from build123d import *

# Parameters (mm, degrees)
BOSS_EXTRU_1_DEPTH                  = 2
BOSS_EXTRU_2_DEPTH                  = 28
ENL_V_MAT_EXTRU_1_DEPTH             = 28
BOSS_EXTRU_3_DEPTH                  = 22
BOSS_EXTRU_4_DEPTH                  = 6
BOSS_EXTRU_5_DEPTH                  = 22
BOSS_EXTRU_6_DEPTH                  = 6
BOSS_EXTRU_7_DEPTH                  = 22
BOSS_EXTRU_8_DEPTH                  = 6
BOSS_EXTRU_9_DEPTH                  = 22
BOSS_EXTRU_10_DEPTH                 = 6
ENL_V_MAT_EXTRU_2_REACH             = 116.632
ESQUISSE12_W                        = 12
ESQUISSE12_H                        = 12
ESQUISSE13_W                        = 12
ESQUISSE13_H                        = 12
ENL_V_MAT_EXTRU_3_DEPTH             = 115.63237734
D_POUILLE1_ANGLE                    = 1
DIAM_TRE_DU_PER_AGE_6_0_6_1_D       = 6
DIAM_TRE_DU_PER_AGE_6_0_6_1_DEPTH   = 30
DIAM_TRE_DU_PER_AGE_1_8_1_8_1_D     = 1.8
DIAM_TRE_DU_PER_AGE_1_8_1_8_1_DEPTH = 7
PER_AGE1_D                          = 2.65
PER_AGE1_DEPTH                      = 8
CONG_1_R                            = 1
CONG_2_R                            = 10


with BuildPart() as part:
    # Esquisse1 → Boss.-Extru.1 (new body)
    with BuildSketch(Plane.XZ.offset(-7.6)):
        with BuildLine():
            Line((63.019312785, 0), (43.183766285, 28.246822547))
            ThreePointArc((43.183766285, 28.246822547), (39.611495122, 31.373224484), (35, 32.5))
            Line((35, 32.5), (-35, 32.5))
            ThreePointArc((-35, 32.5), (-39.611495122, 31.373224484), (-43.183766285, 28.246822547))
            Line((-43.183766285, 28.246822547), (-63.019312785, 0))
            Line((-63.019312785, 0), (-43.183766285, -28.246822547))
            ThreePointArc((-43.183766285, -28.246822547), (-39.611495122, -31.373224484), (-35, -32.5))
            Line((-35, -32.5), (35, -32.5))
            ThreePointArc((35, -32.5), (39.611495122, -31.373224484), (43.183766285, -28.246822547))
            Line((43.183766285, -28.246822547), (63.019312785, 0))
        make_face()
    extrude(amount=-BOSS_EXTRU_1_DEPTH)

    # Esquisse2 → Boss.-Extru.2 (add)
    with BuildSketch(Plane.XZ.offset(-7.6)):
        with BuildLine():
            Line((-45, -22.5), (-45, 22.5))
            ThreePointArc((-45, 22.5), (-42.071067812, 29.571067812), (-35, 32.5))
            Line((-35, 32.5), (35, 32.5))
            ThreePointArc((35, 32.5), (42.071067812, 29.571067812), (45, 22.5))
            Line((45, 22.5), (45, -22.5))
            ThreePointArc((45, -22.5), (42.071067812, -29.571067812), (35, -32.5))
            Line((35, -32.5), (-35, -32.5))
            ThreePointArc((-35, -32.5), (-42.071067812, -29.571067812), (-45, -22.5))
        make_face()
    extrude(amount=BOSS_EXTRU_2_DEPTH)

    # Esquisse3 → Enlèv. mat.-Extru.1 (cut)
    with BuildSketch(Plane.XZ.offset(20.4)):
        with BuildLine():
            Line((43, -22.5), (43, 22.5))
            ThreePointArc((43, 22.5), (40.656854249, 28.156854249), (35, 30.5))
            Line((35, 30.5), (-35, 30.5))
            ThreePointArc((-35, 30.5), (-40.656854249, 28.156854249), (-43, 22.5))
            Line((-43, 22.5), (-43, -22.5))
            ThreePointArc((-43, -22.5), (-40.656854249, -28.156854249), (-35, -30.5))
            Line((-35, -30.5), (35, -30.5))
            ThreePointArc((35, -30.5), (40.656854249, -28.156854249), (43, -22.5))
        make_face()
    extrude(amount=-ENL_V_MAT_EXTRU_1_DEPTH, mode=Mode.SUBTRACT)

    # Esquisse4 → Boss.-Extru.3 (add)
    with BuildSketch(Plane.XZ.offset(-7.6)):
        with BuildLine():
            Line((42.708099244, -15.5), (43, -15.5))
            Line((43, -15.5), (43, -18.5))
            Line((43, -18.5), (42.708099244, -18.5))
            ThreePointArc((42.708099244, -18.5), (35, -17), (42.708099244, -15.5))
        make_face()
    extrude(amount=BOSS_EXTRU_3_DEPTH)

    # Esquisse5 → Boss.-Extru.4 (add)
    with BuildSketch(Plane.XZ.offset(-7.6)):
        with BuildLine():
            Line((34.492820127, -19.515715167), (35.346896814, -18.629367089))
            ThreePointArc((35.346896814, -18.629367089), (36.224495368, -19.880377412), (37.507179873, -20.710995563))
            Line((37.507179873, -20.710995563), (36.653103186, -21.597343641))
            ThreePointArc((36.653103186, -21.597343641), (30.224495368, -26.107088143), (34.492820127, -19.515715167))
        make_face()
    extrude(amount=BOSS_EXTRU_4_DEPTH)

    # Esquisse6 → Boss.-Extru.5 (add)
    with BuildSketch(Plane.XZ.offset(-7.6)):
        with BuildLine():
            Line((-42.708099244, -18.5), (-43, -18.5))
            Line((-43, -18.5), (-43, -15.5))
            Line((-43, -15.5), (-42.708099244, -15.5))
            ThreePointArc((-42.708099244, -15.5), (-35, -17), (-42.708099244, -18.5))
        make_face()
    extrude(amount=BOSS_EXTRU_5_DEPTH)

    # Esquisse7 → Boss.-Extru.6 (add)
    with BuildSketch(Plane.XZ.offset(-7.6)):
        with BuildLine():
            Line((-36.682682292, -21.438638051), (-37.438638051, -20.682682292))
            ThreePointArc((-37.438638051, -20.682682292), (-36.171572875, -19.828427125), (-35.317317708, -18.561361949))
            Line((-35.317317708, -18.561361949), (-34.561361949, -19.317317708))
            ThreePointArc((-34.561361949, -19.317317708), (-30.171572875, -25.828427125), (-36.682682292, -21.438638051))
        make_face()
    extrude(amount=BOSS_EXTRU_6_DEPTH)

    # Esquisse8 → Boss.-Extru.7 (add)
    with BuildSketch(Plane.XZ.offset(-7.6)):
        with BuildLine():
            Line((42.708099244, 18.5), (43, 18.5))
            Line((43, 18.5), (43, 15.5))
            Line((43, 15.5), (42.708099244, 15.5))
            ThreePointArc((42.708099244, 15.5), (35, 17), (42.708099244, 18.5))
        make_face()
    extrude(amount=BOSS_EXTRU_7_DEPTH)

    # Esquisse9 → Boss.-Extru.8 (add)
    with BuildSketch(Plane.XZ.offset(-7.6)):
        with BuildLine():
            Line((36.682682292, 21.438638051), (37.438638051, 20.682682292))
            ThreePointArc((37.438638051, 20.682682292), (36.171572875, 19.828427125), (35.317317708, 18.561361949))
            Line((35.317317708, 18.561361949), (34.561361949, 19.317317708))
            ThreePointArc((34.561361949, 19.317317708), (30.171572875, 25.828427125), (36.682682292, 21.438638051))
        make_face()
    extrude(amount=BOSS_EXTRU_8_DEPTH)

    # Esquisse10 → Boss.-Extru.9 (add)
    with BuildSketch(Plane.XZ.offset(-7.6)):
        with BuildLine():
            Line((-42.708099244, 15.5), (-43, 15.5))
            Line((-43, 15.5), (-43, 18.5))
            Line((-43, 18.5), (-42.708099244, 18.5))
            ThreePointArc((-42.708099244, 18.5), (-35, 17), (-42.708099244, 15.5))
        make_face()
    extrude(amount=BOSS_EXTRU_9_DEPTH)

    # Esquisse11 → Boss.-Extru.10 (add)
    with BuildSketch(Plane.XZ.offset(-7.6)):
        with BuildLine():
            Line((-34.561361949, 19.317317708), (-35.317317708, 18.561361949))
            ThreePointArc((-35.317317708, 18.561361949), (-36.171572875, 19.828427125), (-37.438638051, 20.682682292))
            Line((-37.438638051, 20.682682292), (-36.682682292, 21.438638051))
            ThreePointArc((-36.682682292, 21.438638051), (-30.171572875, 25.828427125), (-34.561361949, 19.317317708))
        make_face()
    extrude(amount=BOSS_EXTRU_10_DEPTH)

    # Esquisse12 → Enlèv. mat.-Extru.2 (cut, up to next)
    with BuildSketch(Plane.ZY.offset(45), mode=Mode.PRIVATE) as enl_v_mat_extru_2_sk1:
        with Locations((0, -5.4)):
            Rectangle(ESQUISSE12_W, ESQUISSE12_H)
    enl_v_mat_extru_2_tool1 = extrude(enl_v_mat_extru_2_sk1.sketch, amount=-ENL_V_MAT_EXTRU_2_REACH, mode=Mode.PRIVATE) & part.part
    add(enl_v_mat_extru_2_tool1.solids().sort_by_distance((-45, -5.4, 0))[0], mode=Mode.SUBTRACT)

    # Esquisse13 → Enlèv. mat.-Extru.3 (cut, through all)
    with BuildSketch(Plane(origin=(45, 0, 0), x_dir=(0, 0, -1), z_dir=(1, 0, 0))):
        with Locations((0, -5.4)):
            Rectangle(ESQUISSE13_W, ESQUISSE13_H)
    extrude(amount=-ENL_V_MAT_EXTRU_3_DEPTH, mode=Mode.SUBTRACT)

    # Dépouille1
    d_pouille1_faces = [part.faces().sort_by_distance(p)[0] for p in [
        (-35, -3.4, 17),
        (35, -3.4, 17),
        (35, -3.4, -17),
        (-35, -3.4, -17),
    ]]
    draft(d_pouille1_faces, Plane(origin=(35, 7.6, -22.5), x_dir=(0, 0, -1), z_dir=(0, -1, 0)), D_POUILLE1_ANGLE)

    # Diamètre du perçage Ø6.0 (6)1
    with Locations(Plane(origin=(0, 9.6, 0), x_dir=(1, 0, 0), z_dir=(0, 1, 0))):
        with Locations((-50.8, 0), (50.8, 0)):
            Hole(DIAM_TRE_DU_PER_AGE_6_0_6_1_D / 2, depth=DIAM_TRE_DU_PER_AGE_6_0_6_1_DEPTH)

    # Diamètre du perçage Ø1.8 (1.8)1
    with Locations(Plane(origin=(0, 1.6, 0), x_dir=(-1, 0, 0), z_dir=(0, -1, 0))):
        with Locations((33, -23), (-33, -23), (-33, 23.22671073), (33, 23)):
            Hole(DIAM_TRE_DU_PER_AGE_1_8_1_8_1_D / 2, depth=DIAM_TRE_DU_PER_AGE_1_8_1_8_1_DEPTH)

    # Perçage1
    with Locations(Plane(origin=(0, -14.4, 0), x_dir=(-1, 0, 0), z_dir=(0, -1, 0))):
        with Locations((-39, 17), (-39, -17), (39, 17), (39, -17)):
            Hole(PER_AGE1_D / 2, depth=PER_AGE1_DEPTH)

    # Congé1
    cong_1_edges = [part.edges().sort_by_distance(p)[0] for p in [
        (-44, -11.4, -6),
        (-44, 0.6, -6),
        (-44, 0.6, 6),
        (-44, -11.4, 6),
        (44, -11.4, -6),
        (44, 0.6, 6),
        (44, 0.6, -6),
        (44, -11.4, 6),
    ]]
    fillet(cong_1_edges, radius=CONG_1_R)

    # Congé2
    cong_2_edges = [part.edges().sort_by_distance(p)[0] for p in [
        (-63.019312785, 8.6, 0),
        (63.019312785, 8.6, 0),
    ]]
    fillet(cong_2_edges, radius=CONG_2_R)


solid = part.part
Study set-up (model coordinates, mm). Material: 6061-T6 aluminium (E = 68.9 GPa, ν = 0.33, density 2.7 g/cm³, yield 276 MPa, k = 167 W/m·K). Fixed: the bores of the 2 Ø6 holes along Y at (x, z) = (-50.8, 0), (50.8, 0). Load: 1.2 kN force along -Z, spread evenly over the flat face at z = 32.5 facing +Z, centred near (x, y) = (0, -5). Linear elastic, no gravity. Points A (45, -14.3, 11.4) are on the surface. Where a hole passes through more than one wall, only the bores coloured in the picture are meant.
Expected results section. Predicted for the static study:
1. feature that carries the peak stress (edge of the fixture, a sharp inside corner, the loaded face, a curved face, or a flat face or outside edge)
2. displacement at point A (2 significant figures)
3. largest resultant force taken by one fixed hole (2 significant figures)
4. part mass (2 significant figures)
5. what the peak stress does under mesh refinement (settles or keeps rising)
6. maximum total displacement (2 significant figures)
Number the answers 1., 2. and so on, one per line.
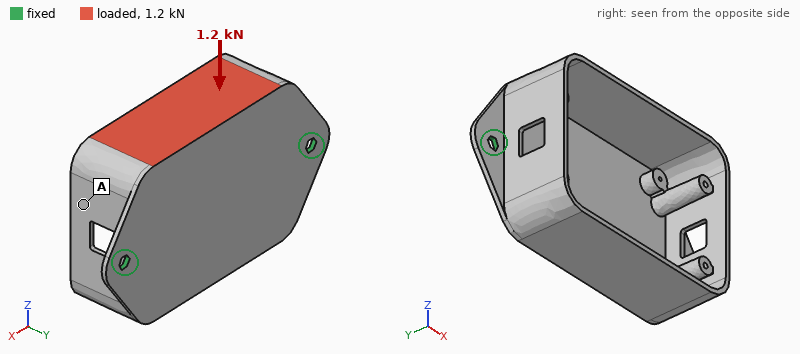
1. edge of the fixture
2. 0.34 mm
3. 600 N
4. 91 g
5. keeps rising
6. 1.3 mm
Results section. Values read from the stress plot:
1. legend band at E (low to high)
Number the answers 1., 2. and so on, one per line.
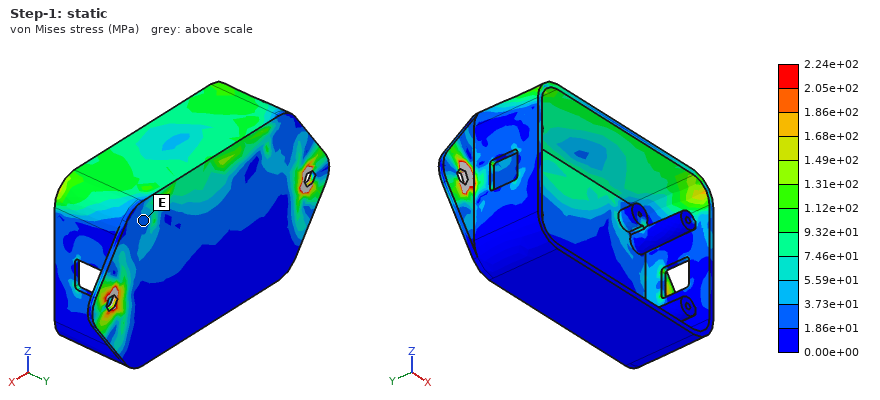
1. 1.86e+01 to 3.73e+01 MPa
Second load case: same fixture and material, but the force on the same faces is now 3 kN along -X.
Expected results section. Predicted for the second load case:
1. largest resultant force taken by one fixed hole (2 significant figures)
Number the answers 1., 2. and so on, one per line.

1. 1.8 kN
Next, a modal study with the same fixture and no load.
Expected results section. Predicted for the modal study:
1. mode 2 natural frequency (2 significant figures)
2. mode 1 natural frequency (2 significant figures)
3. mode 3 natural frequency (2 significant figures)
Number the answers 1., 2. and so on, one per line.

1. 1500 Hz
2. 750 Hz
3. 2300 Hz
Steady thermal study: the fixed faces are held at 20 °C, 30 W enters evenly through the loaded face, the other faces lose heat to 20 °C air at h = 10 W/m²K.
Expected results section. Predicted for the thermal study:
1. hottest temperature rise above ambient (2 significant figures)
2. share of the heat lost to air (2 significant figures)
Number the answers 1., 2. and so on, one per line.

1. 45 K
2. 18 %
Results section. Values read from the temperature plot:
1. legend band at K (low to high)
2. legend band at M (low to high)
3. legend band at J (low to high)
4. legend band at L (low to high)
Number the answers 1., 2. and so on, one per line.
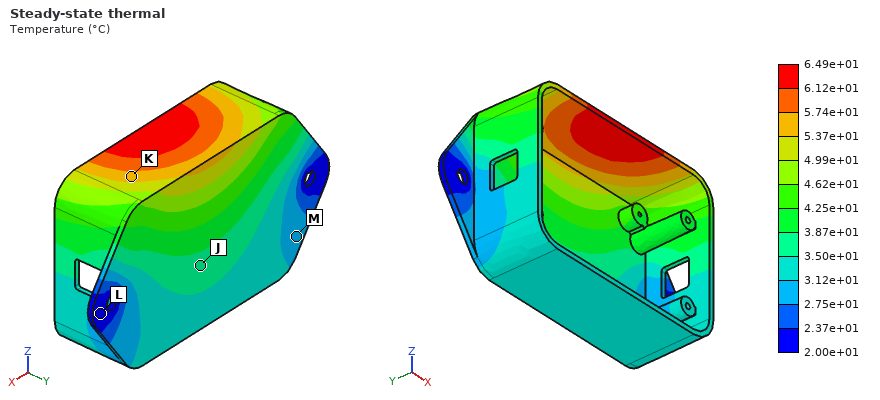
1. 5.37e+01 to 5.74e+01 °C
2. 2.75e+01 to 3.12e+01 °C
3. 3.50e+01 to 3.87e+01 °C
4. 2.00e+01 to 2.37e+01 °C
